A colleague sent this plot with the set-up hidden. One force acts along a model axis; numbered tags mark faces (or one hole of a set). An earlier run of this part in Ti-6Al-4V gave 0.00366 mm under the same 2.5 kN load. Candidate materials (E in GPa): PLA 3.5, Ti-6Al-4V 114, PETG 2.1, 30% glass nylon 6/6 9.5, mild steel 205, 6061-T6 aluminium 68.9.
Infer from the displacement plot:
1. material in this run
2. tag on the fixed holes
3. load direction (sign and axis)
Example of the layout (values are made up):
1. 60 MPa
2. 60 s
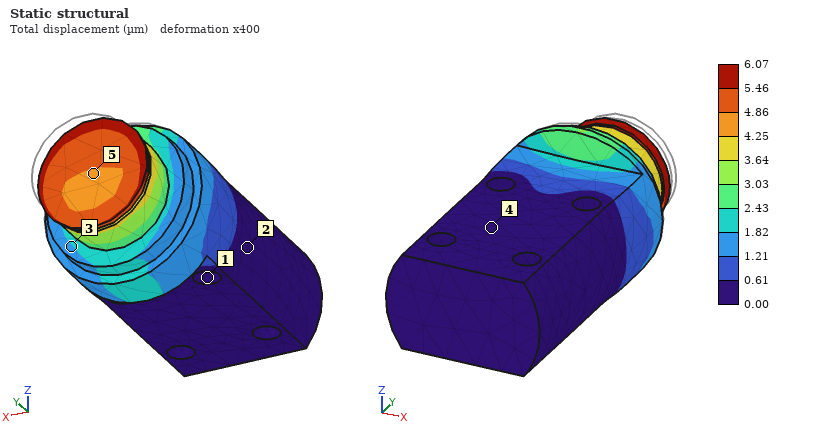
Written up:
1. 6061-T6 aluminium
2. 1
3. -Y
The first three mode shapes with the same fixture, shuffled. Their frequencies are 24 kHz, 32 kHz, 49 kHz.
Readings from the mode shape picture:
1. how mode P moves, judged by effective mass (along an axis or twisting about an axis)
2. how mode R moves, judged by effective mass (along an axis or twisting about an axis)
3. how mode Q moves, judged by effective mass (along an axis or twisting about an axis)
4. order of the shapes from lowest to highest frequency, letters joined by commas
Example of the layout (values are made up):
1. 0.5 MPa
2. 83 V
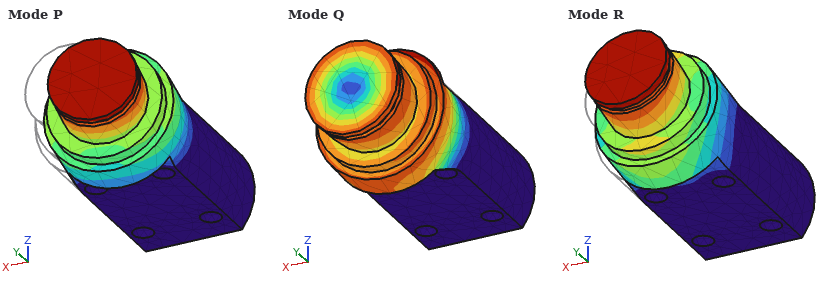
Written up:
1. along X
2. along Z
3. twisting about Y
4. R, P, Q
